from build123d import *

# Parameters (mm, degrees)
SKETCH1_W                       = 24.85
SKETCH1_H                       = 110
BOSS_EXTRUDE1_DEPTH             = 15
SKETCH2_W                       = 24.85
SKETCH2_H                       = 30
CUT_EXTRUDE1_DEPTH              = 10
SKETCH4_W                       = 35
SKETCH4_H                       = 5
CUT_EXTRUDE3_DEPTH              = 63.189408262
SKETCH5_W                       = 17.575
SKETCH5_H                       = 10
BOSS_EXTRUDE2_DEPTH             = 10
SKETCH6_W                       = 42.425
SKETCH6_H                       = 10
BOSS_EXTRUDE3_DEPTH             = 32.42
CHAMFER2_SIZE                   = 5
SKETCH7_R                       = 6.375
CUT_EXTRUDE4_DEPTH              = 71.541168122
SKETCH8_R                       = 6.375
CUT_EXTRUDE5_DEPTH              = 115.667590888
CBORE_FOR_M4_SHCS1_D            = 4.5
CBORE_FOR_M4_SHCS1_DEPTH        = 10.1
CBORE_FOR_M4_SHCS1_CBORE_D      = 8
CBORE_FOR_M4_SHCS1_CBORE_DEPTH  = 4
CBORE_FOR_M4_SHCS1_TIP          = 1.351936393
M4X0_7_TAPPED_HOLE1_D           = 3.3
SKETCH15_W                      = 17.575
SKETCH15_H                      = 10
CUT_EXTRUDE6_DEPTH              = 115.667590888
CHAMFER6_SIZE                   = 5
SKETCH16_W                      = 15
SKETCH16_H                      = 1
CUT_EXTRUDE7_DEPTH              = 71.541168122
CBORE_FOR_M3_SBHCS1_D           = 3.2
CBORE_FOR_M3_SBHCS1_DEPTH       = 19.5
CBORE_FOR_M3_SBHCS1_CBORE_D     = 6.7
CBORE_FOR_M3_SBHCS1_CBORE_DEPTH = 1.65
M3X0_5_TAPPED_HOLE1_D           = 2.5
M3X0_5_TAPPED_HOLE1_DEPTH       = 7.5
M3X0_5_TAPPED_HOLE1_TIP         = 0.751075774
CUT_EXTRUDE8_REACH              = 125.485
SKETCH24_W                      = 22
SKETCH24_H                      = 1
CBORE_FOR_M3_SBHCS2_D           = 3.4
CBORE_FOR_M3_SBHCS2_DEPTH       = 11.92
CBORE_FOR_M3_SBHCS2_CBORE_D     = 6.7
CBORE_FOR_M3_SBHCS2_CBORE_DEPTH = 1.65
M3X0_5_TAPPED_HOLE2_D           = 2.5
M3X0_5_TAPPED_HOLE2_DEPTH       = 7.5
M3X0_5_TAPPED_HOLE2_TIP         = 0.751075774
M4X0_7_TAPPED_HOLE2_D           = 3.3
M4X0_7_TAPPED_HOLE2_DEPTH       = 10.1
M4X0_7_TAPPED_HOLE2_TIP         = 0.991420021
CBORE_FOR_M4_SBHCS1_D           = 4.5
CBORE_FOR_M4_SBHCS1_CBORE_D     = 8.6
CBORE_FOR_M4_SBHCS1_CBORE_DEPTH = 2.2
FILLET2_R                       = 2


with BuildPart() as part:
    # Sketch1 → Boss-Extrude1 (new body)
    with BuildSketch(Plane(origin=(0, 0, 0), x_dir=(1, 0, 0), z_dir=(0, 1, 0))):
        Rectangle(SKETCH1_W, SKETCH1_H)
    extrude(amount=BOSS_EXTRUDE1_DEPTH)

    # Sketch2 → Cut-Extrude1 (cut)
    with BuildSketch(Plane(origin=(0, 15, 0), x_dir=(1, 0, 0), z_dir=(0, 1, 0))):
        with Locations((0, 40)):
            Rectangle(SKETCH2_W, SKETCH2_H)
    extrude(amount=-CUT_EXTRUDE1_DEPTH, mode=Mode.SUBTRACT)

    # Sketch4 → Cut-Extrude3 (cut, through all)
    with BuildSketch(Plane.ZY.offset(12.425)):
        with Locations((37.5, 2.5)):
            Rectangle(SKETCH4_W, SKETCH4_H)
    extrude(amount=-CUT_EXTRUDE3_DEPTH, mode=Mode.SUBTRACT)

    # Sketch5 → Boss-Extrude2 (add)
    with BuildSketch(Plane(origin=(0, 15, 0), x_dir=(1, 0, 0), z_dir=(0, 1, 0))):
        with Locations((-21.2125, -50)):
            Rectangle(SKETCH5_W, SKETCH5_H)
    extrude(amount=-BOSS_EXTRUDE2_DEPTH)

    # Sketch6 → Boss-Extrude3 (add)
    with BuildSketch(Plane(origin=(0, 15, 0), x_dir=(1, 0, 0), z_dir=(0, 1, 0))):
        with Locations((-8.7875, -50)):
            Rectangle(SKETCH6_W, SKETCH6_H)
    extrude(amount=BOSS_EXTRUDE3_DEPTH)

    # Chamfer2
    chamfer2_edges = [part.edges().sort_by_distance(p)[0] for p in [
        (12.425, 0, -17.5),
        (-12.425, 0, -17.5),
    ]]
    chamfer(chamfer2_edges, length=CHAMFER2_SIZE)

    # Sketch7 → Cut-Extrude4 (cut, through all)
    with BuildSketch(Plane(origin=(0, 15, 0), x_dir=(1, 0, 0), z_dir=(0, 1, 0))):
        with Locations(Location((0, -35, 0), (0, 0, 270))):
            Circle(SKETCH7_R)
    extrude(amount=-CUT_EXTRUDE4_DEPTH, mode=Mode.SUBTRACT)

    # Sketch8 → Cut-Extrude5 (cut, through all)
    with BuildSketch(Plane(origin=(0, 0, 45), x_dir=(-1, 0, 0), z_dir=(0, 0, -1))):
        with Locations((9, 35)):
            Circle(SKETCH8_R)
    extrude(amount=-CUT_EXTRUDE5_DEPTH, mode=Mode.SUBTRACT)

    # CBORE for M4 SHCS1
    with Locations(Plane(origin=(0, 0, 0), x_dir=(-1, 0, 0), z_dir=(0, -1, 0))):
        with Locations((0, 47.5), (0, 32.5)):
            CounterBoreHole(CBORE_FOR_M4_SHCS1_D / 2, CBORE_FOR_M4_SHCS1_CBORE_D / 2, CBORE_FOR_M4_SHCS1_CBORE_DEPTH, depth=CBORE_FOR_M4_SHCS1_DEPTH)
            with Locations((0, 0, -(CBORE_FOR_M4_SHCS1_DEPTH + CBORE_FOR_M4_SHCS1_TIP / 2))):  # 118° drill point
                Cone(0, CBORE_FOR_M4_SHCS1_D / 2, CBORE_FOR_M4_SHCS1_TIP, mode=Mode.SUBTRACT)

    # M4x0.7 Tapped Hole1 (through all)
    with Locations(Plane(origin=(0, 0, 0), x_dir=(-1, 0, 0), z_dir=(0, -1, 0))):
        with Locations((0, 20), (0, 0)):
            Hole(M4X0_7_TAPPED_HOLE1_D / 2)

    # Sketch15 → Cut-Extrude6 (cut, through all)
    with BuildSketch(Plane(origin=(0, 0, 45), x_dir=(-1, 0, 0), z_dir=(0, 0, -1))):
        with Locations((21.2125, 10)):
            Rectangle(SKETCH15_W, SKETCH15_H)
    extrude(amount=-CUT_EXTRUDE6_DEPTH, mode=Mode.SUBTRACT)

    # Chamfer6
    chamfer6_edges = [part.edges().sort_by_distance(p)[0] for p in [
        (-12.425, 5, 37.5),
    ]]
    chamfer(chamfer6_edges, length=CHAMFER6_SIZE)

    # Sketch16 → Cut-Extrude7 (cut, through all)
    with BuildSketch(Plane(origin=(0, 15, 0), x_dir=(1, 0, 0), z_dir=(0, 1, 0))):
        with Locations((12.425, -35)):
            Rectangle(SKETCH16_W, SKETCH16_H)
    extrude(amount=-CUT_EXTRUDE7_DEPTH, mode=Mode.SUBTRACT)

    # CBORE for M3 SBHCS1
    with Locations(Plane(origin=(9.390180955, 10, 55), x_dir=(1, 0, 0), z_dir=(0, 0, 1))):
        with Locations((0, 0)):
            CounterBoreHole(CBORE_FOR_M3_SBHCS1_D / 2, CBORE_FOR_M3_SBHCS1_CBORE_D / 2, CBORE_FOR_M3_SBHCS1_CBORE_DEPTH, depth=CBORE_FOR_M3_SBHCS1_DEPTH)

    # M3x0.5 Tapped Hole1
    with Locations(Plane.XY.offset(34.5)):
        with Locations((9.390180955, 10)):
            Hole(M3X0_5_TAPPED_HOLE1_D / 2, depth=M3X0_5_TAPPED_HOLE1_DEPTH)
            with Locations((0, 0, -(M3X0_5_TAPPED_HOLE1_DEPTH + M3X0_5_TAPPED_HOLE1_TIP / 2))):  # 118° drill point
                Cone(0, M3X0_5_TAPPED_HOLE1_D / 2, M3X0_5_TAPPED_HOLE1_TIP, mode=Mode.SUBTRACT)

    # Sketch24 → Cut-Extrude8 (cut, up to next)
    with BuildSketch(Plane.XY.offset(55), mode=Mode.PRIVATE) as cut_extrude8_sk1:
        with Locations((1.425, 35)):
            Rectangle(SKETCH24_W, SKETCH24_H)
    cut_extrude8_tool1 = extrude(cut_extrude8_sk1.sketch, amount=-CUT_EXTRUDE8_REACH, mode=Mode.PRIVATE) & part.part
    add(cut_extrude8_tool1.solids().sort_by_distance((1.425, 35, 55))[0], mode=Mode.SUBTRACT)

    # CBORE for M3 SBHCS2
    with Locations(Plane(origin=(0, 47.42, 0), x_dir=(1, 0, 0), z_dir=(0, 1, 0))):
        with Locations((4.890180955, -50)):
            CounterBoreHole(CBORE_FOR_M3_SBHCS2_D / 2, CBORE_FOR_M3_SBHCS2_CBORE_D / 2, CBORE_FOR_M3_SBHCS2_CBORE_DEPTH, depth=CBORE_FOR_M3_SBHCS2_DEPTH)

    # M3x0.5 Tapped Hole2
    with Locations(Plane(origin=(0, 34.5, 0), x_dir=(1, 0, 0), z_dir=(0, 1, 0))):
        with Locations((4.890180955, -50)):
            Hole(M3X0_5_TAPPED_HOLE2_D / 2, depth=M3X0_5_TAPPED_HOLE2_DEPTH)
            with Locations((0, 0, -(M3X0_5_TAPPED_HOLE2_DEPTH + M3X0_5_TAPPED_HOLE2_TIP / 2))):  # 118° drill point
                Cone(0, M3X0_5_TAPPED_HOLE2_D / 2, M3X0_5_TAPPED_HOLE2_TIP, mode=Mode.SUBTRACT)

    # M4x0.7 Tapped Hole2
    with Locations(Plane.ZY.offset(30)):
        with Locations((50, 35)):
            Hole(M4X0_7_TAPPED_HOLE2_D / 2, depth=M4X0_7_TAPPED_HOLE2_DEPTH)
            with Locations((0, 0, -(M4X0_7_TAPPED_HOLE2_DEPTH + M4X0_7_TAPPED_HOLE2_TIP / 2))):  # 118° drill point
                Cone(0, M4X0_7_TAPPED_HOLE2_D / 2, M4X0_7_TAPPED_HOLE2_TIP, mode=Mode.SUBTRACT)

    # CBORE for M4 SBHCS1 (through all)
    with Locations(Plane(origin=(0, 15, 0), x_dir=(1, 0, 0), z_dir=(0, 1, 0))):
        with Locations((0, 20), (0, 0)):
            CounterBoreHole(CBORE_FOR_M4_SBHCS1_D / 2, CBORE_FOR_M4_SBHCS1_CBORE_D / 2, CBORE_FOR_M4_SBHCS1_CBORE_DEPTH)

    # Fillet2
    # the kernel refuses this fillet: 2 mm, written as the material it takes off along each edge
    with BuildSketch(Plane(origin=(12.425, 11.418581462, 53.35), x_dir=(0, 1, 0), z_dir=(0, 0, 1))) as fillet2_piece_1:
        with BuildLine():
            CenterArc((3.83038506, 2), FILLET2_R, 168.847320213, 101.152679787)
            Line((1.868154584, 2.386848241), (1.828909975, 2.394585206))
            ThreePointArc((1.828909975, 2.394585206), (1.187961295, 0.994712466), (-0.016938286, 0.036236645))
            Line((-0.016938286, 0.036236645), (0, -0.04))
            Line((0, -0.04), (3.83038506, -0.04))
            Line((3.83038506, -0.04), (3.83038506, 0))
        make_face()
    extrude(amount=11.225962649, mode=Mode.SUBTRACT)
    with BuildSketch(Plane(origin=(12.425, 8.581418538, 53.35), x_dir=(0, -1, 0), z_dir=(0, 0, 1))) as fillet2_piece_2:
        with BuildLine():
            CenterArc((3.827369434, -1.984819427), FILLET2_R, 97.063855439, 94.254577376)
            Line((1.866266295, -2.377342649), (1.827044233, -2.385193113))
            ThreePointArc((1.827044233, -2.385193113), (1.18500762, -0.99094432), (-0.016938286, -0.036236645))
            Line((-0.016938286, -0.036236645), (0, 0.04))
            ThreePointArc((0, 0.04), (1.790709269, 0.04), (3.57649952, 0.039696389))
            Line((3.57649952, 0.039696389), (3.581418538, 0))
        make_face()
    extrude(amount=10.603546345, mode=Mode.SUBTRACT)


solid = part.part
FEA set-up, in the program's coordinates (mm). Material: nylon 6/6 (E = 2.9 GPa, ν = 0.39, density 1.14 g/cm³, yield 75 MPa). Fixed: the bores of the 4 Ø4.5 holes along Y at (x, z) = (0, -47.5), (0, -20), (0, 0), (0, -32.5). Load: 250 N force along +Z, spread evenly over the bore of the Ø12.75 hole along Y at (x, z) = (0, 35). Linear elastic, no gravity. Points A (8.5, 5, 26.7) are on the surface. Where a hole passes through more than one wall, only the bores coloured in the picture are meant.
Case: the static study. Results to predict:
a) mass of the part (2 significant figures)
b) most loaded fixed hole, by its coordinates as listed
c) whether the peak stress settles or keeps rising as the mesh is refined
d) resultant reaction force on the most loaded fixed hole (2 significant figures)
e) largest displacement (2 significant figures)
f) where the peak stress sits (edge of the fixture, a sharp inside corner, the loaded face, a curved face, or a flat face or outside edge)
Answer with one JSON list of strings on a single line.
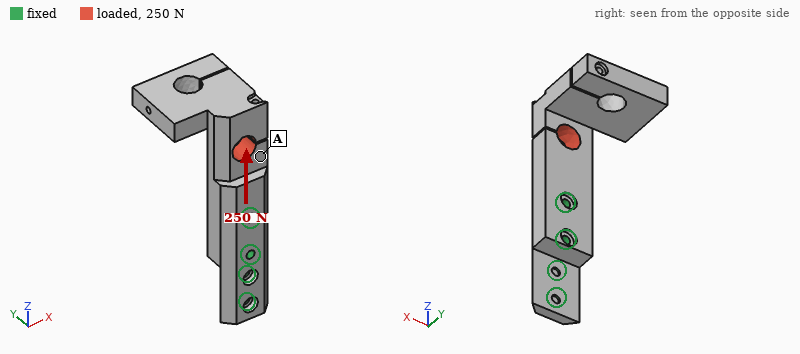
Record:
["41 g", "(0, 0)", "keeps rising", "200 N", "1.1 mm", "a sharp inside corner"]
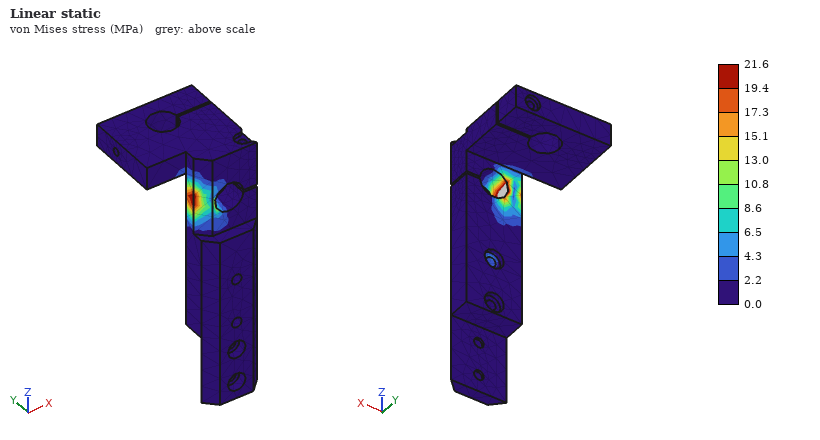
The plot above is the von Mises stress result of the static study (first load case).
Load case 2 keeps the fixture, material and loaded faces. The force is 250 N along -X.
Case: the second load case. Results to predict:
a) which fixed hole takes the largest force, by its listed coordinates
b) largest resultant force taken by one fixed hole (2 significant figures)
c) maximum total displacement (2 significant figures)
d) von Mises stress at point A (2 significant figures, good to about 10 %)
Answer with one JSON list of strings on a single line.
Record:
["(0, 0)", "560 N", "0.94 mm", "1.1 MPa"]
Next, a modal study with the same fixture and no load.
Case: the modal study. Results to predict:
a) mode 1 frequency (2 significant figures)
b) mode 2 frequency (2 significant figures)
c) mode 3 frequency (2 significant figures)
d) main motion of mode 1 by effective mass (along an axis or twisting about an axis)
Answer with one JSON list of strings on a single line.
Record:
["230 Hz", "290 Hz", "440 Hz", "along X"]
